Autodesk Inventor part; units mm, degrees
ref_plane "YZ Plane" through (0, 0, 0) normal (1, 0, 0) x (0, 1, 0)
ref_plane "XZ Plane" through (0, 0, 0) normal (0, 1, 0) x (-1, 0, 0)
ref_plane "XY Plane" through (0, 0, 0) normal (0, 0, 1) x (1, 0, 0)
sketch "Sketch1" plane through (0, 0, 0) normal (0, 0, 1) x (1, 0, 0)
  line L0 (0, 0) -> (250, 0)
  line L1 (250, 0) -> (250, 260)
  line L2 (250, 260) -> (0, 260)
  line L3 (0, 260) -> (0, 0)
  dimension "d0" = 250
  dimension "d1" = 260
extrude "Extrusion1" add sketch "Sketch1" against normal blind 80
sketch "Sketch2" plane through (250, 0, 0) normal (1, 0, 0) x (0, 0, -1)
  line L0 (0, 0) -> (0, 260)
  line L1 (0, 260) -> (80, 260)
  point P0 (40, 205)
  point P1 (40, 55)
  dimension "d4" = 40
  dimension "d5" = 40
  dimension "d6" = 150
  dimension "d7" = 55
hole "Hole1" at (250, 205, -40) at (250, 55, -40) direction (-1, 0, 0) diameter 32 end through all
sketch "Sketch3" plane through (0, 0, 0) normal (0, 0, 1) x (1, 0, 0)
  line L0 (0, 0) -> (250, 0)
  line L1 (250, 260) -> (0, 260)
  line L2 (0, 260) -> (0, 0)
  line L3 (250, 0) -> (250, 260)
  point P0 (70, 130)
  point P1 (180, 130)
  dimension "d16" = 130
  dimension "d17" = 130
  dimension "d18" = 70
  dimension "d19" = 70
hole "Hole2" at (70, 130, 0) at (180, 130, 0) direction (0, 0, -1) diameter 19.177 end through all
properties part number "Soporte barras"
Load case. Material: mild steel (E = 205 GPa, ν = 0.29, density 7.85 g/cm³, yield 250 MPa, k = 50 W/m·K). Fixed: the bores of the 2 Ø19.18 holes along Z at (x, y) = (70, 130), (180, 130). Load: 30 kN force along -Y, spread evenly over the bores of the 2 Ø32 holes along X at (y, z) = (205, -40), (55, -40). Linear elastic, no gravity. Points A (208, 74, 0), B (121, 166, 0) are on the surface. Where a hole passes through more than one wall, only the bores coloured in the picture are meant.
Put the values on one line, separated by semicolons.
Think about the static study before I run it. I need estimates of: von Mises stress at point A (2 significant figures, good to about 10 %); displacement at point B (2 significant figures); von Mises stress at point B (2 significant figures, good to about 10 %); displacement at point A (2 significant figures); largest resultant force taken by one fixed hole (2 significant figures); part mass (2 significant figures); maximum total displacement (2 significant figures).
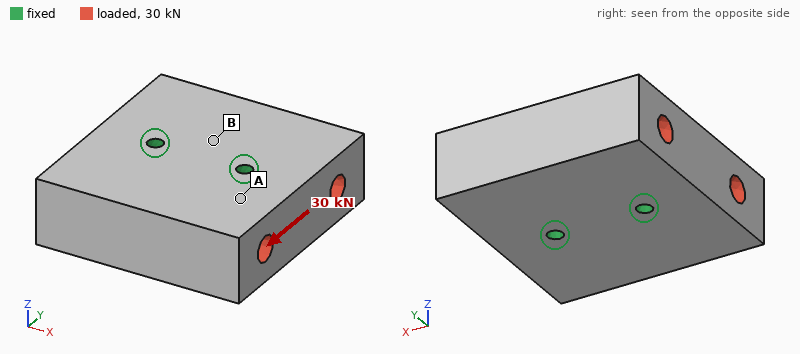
0.85 MPa; 0.39 µm; 0.39 MPa; 0.51 µm; 15 kN; 37 kg; 0.75 µm
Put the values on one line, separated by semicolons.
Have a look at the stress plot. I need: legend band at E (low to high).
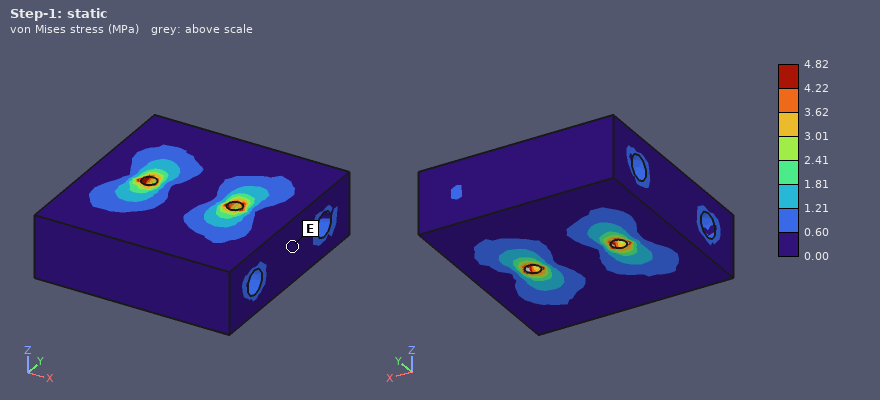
0.00 to 0.60 MPa
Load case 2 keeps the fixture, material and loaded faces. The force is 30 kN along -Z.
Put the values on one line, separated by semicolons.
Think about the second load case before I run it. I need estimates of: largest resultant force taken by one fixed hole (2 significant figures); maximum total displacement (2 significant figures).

15 kN; 3.4 µm
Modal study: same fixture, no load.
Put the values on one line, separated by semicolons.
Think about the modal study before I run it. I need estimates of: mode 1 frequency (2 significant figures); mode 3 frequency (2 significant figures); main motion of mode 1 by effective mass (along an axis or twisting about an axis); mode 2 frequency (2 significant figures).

2200 Hz; 3000 Hz; twisting about X; 3000 Hz
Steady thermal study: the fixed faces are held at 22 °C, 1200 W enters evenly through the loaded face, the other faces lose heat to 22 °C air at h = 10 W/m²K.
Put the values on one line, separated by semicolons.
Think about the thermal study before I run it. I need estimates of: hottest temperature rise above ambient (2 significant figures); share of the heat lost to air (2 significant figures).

69 K; 8.8 %
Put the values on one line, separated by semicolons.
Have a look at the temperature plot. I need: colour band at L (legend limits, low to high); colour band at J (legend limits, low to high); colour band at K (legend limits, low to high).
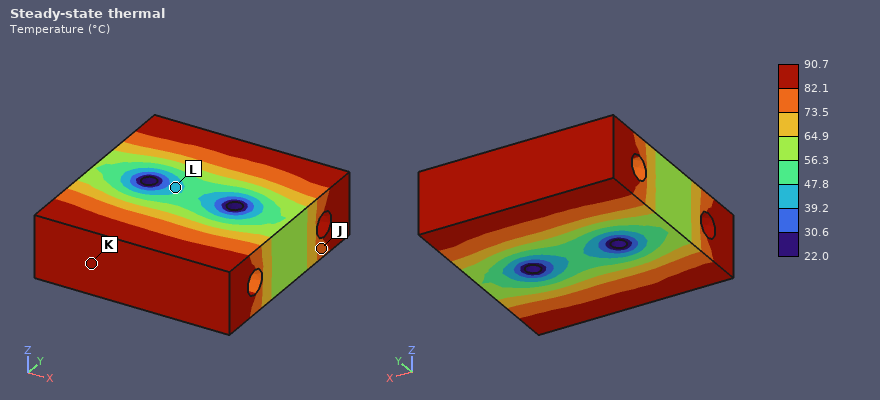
39.2 to 47.8 °C; 73.5 to 82.1 °C; 82.1 to 90.7 °C
